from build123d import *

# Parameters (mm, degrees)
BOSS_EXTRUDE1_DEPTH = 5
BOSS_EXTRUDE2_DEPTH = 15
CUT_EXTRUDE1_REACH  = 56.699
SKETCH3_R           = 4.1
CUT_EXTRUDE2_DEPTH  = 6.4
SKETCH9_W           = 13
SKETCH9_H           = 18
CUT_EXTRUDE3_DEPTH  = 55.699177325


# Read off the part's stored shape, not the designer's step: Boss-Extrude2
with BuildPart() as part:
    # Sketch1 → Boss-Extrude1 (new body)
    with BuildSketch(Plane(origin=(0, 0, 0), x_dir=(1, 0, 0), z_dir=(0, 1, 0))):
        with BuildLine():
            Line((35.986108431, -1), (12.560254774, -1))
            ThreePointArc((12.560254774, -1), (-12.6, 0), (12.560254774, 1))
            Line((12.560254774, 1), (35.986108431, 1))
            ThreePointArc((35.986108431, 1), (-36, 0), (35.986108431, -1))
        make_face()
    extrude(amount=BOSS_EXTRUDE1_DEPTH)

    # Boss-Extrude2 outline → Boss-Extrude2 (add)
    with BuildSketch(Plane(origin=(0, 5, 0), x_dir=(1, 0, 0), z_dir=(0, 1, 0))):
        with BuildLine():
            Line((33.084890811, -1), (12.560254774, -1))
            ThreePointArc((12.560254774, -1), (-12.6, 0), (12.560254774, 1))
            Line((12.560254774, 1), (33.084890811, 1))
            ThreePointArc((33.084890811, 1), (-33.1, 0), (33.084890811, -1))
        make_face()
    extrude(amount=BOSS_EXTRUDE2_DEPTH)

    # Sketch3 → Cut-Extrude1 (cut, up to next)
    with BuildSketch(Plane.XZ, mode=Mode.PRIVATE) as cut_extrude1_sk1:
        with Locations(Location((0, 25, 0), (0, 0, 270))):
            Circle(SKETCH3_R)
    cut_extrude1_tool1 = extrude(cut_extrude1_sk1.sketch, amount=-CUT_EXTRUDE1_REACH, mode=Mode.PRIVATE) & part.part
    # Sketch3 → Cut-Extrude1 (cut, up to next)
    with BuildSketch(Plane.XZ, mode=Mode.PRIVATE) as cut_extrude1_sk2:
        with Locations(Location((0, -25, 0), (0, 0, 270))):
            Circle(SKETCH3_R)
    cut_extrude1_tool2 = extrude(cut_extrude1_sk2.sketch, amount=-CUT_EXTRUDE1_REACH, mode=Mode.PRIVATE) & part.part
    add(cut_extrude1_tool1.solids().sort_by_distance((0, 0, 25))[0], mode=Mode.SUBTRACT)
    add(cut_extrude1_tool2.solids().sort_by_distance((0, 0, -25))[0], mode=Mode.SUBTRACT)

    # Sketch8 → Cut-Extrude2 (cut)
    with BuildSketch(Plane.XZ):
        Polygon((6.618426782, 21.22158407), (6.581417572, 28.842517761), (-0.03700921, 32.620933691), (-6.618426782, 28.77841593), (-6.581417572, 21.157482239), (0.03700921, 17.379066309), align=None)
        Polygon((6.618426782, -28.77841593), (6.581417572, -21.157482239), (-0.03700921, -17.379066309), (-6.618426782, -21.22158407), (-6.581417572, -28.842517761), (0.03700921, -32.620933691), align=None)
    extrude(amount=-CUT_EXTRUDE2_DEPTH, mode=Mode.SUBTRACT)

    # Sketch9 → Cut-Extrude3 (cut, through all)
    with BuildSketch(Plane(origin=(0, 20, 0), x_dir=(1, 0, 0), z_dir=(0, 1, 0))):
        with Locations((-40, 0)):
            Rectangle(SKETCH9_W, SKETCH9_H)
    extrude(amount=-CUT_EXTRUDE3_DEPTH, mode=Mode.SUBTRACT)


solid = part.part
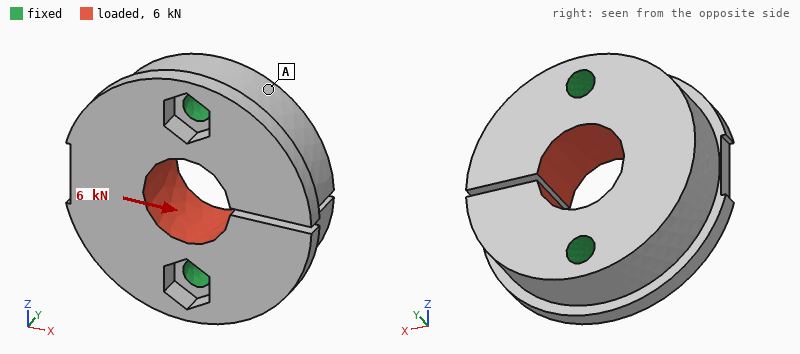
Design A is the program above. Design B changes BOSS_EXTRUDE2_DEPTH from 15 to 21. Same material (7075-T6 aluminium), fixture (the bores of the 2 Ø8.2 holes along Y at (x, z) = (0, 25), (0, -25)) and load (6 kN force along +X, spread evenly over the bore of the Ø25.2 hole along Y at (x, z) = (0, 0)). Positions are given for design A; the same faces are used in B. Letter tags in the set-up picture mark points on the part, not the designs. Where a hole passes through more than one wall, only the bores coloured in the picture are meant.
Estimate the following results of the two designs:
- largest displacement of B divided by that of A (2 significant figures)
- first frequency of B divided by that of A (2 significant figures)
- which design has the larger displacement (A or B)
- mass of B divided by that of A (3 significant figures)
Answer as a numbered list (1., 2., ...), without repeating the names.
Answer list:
1. 0.73
2. 1.2
3. A
4. 1.29
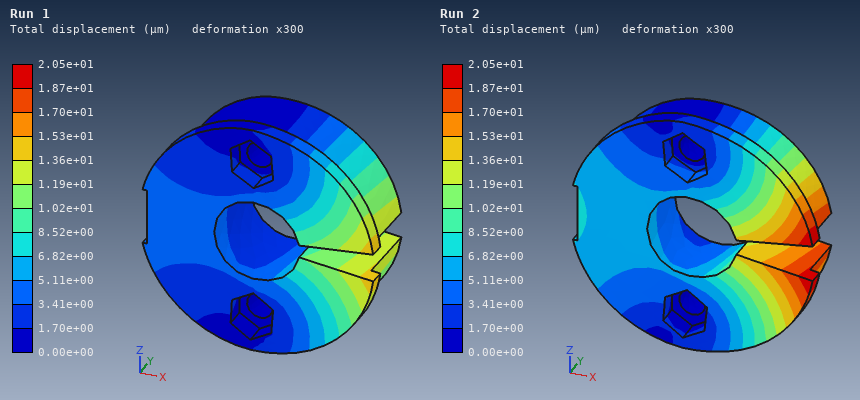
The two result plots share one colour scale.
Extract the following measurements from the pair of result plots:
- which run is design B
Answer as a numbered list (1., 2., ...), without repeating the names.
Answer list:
1. Run 1
